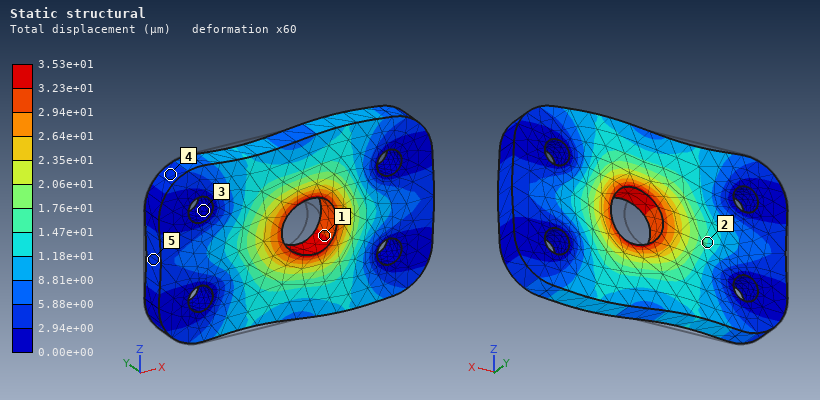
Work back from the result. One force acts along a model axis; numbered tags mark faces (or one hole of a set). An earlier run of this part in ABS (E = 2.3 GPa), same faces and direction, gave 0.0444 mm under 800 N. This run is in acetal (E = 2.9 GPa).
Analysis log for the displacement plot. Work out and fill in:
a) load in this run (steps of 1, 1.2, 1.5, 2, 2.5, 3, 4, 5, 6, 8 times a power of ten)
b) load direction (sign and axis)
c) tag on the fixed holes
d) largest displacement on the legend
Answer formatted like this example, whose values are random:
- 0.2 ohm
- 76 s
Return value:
- 800 N
- +X
- 3
- 3.53e+01 µm
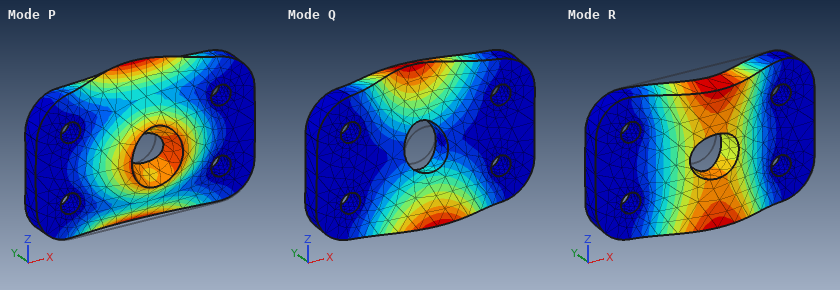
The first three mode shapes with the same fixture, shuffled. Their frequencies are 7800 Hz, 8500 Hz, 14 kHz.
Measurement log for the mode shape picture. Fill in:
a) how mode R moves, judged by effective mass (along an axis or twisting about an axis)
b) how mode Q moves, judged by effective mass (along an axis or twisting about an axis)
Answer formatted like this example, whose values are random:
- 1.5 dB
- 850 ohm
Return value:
- along Y
- twisting about X
